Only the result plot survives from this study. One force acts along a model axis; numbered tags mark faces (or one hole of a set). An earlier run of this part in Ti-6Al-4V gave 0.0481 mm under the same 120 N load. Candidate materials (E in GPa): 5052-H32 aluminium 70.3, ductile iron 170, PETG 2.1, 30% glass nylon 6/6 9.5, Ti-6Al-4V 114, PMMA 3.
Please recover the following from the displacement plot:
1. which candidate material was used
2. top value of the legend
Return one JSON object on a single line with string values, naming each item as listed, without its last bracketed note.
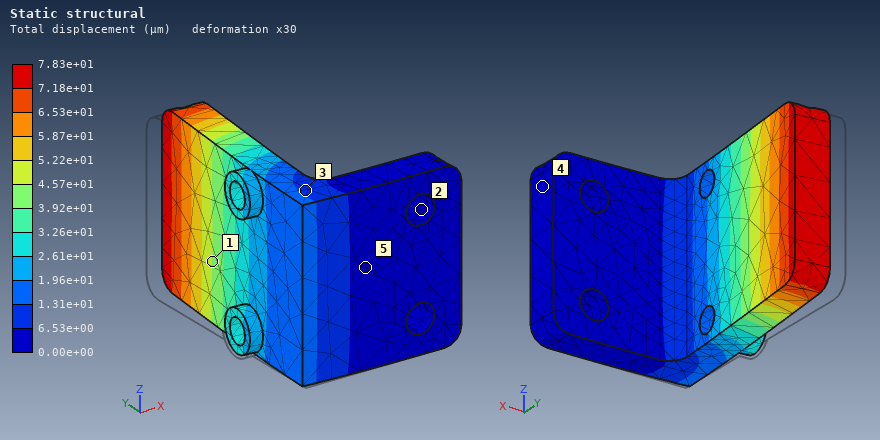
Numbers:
{"which candidate material was used": "5052-H32 aluminium", "top value of the legend": "7.83e+01 µm"}
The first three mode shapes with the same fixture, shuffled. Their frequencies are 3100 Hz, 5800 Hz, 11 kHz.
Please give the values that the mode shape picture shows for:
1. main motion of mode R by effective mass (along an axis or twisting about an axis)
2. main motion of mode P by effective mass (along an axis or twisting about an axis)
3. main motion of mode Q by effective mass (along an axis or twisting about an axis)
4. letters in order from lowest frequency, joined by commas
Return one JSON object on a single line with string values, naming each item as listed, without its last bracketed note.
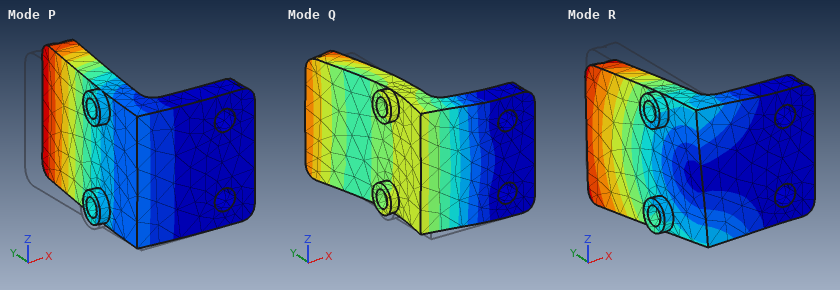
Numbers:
{"main motion of mode R by effective mass": "along Z", "main motion of mode P by effective mass": "along X", "main motion of mode Q by effective mass": "along Y", "letters in order from lowest frequency, joined by commas": "P, R, Q"}
